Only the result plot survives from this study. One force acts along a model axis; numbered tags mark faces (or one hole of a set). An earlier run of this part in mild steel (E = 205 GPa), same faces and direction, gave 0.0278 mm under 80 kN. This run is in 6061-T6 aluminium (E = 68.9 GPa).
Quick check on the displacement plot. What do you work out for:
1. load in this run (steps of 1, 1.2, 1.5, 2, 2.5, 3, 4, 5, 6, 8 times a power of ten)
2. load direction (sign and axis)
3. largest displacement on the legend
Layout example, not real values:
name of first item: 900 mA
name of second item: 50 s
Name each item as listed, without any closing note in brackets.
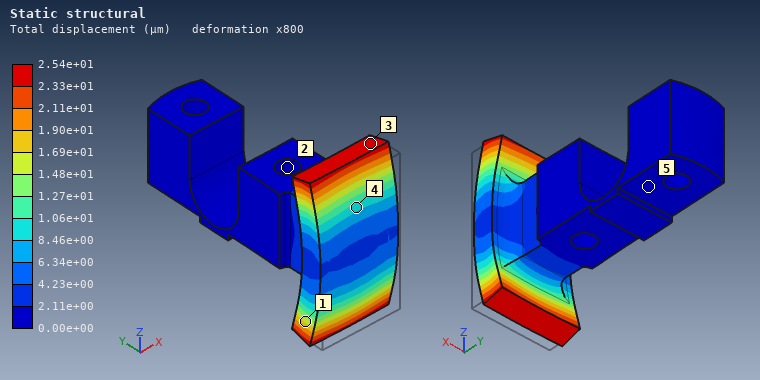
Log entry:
load in this run: 25 kN
load direction: +Y
largest displacement on the legend: 2.54e+01 µm
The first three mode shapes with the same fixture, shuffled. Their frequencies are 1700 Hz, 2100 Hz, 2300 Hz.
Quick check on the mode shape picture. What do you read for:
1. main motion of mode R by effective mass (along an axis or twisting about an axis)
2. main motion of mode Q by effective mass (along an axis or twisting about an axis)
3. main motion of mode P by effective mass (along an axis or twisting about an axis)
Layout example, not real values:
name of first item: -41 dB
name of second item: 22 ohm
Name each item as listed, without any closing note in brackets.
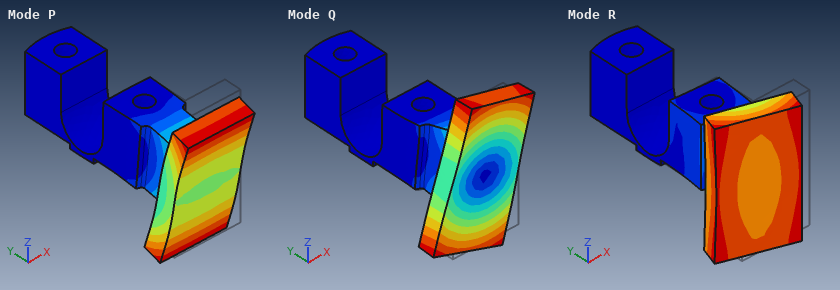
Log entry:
main motion of mode R by effective mass: along X
main motion of mode Q by effective mass: twisting about Y
main motion of mode P by effective mass: along Z
